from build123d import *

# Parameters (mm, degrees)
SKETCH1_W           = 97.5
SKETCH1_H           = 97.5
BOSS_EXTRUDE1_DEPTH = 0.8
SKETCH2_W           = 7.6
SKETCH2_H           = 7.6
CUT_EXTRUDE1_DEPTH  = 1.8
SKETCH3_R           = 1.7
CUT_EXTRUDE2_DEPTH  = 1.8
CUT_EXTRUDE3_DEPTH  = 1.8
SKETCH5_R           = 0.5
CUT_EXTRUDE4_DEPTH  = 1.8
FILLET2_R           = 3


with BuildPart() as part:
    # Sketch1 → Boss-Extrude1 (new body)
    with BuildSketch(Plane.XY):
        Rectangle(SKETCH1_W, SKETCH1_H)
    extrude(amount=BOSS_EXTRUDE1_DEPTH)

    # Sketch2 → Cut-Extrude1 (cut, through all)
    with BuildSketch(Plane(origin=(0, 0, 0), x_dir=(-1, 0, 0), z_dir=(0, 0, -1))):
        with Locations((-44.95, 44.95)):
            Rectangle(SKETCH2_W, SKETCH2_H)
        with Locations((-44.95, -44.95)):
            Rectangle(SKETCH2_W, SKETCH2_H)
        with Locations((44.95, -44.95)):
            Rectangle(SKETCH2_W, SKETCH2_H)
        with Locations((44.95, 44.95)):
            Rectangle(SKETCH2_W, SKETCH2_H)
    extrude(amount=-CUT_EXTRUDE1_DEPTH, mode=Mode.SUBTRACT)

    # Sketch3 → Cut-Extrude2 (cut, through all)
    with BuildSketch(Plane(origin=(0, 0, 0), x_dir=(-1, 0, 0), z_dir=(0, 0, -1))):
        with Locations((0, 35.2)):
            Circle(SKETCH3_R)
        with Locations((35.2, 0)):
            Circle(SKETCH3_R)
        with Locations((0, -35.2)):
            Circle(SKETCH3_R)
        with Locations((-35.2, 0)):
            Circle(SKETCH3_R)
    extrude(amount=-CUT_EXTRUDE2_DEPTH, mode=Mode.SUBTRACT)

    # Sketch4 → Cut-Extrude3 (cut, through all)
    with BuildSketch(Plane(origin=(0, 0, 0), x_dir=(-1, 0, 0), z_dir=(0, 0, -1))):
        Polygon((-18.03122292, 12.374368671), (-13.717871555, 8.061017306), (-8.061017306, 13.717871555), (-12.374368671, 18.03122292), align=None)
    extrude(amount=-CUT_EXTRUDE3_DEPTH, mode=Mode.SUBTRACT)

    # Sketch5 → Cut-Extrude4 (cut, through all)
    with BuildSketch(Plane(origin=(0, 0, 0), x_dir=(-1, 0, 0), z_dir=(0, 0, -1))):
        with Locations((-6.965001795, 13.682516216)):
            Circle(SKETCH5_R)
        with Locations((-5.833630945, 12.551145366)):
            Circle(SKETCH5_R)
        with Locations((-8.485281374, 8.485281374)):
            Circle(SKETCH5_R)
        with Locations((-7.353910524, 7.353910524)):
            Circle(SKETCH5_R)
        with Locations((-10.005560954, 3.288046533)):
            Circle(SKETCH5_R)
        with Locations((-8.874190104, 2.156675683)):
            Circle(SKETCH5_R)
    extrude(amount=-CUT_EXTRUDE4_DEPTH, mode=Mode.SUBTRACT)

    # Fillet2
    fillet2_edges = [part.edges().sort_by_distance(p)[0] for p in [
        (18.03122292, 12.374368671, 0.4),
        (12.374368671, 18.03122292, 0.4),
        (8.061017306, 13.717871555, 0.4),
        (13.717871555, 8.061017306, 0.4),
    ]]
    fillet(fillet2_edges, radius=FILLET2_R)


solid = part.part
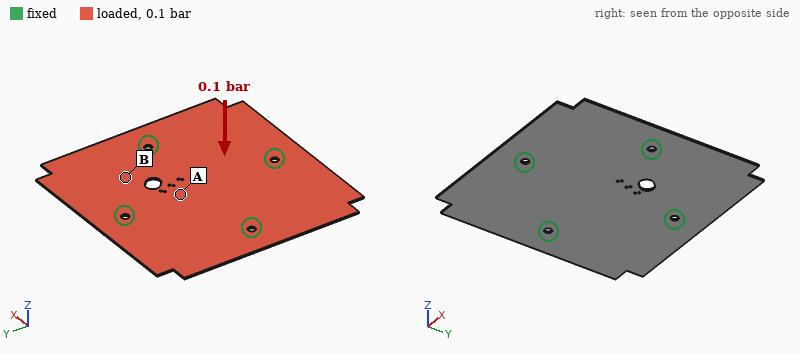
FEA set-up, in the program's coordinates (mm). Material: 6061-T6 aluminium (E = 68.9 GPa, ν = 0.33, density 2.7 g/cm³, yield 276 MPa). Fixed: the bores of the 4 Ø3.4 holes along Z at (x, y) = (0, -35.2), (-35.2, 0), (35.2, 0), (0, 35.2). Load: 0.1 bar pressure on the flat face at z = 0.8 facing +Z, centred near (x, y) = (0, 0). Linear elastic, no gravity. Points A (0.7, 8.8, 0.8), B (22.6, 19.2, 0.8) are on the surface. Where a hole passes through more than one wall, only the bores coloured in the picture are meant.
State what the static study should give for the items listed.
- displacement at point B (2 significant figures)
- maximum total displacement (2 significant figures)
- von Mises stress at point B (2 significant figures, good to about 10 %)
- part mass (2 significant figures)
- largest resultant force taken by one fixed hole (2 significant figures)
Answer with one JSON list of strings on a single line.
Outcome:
["0.098 mm", "0.55 mm", "18 MPa", "20 g", "23 N"]
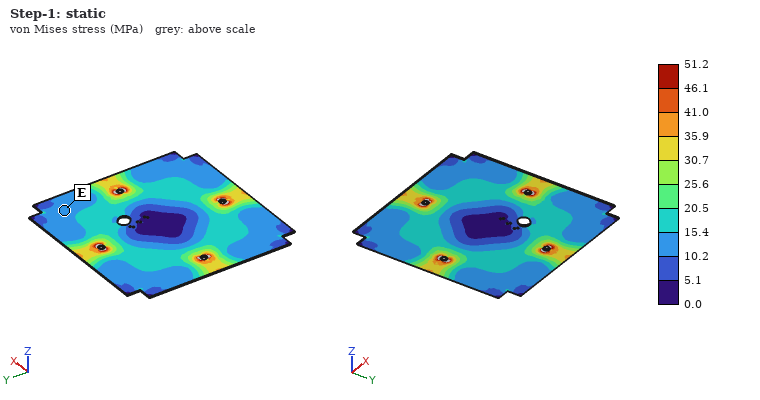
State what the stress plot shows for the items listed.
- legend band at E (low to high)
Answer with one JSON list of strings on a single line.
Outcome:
["10.2 to 15.4 MPa"]
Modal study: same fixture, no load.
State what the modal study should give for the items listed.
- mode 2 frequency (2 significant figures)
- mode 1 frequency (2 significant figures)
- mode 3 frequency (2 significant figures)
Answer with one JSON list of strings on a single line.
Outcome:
["600 Hz", "560 Hz", "600 Hz"]
